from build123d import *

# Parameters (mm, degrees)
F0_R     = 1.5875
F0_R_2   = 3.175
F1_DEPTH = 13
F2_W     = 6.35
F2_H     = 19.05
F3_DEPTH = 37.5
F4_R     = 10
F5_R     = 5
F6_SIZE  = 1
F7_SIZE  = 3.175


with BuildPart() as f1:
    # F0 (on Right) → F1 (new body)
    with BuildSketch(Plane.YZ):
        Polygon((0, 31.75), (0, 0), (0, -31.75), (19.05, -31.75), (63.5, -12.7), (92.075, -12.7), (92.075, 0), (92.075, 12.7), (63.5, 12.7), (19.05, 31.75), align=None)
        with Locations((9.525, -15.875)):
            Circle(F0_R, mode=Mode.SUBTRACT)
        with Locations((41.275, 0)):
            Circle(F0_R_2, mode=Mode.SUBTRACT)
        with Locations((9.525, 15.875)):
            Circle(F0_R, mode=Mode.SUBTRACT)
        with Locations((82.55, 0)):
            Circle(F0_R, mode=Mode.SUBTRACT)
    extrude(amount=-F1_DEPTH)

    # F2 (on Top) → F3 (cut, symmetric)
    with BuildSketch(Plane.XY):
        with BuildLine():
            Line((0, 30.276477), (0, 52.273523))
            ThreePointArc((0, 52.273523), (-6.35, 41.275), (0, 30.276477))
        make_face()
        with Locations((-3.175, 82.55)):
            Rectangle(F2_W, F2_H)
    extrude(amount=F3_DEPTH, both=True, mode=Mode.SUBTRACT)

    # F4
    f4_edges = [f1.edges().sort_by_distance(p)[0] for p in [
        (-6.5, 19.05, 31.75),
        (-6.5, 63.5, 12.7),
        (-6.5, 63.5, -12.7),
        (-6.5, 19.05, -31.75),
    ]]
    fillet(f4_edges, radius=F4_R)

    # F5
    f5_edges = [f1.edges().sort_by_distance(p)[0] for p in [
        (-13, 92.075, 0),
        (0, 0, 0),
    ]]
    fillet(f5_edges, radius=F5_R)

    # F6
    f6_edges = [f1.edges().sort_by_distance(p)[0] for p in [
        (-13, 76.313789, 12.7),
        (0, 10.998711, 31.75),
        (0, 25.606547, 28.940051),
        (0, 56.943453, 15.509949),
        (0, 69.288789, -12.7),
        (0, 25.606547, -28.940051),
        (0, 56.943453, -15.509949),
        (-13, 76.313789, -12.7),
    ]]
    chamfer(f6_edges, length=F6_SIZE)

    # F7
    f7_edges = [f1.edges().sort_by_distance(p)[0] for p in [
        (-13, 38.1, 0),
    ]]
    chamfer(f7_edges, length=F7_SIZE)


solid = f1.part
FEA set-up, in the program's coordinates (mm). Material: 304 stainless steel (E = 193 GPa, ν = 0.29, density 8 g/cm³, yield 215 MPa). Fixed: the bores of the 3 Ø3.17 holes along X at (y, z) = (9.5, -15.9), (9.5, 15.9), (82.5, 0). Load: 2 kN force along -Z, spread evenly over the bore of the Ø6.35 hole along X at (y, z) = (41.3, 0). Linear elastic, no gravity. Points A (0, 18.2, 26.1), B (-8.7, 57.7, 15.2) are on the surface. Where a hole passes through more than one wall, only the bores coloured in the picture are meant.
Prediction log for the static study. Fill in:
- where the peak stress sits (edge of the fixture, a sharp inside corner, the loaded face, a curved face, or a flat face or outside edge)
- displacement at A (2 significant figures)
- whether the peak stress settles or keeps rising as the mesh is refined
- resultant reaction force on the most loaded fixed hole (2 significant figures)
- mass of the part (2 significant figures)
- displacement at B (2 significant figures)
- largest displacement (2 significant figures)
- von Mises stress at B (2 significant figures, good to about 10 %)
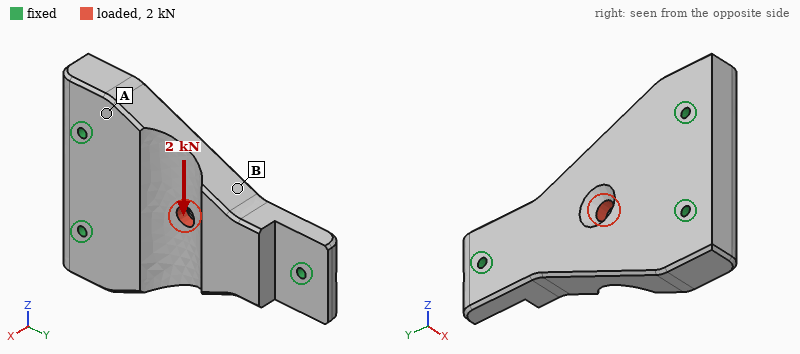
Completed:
a sharp inside corner
0.91 µm
keeps rising
1.3 kN
340 g
2.2 µm
3.1 µm
8.4 MPa
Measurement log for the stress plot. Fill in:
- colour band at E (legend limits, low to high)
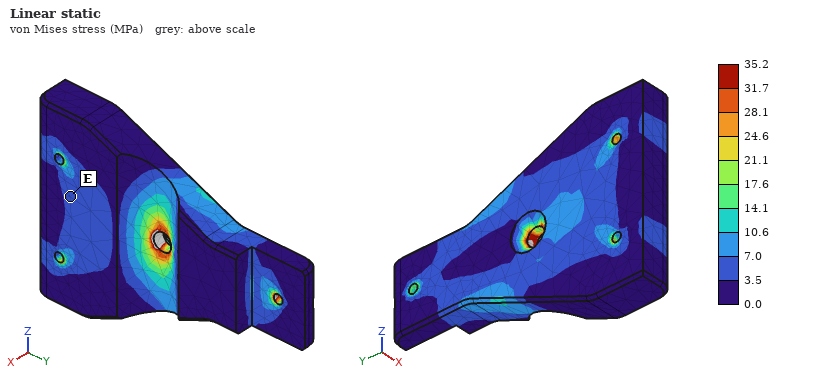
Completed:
3.5 to 7.0 MPa
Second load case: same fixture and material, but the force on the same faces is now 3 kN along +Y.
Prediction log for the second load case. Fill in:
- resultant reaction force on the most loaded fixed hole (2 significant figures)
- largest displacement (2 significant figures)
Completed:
1.1 kN
2.3 µm
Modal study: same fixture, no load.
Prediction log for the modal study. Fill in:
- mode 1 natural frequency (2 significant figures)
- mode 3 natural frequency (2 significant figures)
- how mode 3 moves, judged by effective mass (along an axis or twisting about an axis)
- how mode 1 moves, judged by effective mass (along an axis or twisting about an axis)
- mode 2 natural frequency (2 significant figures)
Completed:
6900 Hz
13 kHz
along Z
along X
9800 Hz
